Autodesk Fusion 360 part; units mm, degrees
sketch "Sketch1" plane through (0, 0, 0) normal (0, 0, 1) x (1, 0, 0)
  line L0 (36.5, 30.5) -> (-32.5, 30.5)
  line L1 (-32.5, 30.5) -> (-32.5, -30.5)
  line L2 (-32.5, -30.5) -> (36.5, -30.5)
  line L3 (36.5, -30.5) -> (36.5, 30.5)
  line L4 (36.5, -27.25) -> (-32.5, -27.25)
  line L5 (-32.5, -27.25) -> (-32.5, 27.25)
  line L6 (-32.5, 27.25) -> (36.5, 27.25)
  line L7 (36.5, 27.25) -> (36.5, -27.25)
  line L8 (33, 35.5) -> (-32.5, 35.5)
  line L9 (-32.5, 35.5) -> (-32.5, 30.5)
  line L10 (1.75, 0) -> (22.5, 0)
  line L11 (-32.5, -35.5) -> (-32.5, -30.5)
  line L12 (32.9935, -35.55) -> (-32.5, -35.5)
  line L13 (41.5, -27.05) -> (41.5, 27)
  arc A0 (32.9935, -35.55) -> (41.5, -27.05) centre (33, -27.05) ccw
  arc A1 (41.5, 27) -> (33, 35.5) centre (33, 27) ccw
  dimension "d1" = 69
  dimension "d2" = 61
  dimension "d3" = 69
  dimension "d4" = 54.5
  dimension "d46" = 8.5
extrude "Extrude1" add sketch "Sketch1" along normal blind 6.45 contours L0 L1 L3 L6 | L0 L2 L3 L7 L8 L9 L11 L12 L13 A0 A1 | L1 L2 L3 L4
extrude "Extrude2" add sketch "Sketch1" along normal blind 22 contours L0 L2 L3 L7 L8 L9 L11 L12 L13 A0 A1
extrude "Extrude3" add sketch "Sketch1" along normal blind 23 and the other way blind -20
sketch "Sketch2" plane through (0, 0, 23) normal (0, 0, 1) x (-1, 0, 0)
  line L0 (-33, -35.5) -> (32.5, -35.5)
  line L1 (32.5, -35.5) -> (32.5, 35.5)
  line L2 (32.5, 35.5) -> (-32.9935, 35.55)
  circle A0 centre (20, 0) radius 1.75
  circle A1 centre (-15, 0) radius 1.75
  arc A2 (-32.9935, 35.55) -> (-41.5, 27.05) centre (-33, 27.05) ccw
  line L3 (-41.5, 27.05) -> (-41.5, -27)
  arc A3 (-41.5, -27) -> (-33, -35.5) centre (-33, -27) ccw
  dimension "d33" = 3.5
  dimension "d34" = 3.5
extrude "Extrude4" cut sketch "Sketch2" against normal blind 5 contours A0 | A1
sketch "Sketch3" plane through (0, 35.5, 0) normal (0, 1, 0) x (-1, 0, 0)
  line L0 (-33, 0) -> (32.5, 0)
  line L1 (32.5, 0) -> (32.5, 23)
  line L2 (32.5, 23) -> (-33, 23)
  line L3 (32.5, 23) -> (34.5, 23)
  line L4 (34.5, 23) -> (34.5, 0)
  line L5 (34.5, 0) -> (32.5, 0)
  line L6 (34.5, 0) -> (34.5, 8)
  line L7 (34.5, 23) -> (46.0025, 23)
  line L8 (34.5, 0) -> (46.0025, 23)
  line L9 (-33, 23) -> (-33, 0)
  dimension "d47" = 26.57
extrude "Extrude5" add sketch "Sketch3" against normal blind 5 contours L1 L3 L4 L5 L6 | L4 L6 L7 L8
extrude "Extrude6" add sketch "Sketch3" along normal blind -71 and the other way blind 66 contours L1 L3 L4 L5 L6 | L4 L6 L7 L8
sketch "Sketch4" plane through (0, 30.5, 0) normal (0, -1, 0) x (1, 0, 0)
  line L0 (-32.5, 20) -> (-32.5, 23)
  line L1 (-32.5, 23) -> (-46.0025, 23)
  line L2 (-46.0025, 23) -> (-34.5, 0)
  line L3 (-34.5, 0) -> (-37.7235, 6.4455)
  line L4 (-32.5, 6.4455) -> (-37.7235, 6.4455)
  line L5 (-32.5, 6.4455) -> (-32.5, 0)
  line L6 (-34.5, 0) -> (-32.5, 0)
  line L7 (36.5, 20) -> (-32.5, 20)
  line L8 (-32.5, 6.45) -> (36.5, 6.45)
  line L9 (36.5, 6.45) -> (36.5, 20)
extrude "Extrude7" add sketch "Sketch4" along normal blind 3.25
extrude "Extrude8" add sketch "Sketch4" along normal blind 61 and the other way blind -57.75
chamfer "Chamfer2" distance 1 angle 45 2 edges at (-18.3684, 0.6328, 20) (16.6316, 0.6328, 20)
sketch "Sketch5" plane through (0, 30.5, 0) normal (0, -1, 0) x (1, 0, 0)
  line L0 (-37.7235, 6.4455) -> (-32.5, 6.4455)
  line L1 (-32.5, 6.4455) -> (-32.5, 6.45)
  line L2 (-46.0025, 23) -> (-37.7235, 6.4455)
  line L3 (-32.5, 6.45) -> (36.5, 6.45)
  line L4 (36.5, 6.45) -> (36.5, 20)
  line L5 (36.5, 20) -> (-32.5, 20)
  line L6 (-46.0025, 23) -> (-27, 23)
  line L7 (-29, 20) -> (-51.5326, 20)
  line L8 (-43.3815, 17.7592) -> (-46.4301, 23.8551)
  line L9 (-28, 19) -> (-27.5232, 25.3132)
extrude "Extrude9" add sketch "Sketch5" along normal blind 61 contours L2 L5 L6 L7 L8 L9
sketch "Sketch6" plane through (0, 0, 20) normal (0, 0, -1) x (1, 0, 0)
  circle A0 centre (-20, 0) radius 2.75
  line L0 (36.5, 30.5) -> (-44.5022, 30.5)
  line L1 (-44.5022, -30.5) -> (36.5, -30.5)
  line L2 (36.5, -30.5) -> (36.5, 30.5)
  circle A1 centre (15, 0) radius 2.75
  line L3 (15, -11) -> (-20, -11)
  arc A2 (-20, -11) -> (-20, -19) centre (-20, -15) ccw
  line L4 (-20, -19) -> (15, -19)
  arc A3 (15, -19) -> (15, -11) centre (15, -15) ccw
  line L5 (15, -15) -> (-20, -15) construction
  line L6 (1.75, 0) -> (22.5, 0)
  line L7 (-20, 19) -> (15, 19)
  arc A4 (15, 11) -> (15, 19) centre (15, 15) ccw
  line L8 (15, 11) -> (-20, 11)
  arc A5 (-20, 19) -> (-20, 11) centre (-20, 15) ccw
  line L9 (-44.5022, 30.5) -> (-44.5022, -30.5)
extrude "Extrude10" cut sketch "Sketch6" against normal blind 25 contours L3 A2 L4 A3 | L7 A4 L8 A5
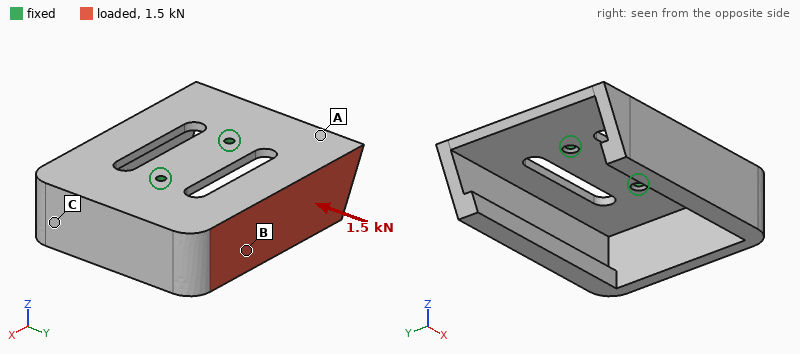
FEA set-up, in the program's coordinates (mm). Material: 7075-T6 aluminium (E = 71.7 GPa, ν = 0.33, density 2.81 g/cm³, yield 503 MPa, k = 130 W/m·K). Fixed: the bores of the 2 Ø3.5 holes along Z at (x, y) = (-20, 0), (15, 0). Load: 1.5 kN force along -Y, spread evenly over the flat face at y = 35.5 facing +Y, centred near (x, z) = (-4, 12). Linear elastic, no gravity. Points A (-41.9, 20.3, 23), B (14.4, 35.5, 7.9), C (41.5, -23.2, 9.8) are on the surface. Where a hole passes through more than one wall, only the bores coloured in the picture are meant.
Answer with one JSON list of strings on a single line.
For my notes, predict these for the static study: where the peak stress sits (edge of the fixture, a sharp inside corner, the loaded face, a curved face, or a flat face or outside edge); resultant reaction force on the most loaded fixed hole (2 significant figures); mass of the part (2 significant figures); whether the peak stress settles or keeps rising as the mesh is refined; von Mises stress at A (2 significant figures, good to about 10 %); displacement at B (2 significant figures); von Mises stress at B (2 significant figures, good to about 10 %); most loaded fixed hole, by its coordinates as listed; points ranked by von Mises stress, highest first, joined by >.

["edge of the fixture", "820 N", "120 g", "keeps rising", "88 MPa", "0.91 mm", "45 MPa", "(-20, 0)", "A > B > C"]
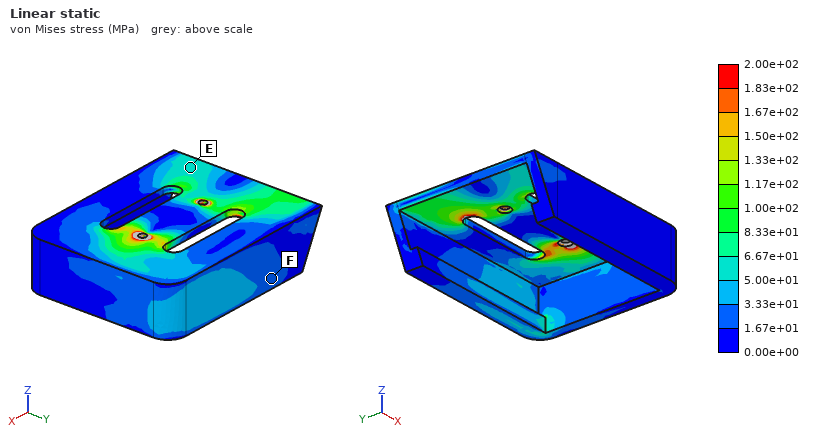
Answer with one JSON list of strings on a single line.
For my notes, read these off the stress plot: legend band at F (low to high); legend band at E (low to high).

["1.67e+01 to 3.33e+01 MPa", "5.00e+01 to 6.67e+01 MPa"]
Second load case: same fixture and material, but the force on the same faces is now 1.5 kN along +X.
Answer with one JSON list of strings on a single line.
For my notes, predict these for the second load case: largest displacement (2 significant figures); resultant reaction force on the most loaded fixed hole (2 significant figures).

["0.31 mm", "1.6 kN"]
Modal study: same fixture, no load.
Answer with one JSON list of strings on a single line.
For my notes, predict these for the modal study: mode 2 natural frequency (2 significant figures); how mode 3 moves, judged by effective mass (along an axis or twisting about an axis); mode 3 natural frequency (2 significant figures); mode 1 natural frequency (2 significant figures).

["1100 Hz", "along Z", "1300 Hz", "470 Hz"]
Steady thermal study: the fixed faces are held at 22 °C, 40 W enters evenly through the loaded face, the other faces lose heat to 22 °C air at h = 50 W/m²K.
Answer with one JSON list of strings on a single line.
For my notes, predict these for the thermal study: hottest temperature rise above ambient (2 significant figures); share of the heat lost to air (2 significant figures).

["53 K", "52 %"]
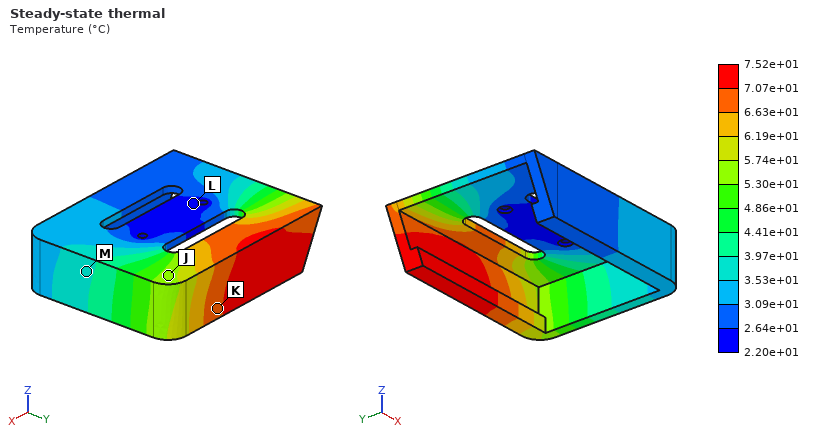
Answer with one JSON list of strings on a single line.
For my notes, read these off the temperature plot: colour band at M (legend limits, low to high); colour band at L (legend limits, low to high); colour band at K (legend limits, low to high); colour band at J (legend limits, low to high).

["3.53e+01 to 3.97e+01 °C", "2.20e+01 to 2.64e+01 °C", "6.63e+01 to 7.07e+01 °C", "5.30e+01 to 5.74e+01 °C"]
